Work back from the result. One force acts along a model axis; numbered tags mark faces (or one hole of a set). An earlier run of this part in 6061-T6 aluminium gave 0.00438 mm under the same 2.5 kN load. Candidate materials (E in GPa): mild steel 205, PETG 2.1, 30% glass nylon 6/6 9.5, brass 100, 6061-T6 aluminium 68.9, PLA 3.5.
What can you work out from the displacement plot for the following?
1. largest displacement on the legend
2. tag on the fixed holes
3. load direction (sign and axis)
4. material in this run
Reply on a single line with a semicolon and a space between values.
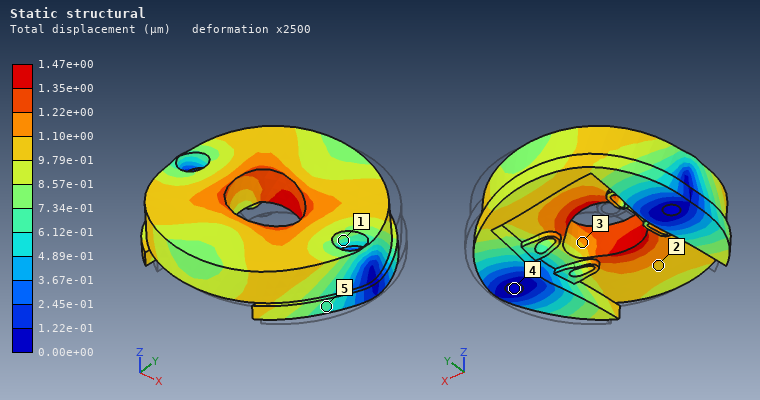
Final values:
1.47e+00 µm; 4; -X; mild steel
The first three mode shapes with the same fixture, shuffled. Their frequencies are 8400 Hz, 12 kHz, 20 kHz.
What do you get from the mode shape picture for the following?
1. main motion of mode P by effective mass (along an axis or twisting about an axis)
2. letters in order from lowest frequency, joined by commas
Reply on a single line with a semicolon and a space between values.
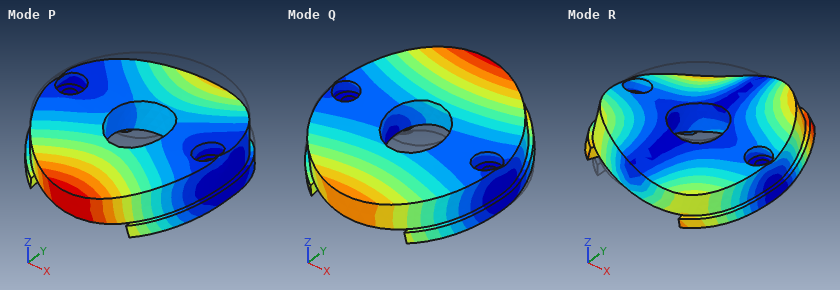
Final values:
along Z; Q, P, R
